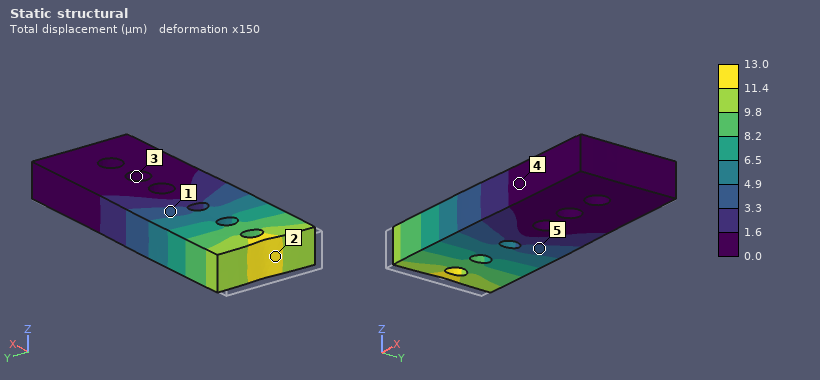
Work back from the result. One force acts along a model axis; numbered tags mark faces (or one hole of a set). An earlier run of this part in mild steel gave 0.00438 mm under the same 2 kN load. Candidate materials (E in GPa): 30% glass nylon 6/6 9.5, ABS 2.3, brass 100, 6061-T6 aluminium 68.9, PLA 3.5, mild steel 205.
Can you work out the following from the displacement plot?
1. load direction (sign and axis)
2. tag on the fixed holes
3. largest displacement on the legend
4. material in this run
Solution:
+X
3
13.0 µm
6061-T6 aluminium
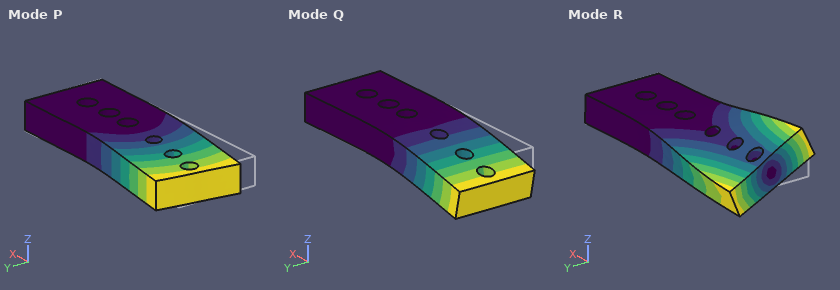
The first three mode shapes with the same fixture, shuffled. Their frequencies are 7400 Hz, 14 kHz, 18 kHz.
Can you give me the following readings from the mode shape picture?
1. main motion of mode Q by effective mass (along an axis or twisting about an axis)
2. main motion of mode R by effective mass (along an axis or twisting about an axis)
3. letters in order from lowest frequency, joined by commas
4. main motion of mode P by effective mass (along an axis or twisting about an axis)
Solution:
along Z
twisting about X
Q, P, R
along Y
